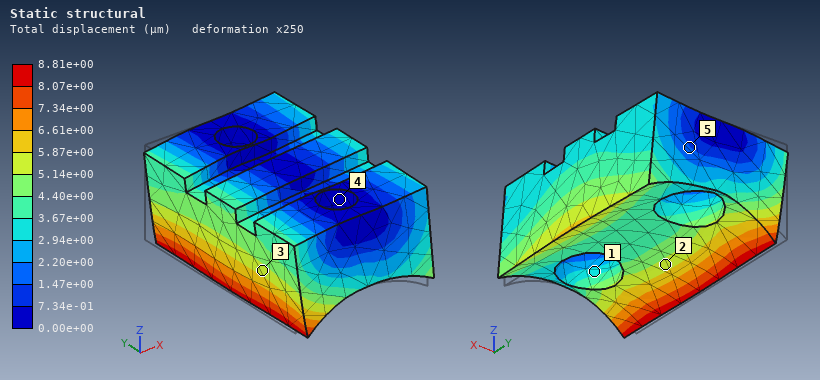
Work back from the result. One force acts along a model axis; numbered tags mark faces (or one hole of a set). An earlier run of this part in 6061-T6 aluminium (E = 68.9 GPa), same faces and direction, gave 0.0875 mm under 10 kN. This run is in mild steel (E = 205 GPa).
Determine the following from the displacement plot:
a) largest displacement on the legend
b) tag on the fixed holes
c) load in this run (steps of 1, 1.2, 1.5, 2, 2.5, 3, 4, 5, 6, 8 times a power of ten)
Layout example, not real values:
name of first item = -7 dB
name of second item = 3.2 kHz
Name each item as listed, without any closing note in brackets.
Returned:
largest displacement on the legend = 8.81e+00 µm
tag on the fixed holes = 4
load in this run = 3 kN
